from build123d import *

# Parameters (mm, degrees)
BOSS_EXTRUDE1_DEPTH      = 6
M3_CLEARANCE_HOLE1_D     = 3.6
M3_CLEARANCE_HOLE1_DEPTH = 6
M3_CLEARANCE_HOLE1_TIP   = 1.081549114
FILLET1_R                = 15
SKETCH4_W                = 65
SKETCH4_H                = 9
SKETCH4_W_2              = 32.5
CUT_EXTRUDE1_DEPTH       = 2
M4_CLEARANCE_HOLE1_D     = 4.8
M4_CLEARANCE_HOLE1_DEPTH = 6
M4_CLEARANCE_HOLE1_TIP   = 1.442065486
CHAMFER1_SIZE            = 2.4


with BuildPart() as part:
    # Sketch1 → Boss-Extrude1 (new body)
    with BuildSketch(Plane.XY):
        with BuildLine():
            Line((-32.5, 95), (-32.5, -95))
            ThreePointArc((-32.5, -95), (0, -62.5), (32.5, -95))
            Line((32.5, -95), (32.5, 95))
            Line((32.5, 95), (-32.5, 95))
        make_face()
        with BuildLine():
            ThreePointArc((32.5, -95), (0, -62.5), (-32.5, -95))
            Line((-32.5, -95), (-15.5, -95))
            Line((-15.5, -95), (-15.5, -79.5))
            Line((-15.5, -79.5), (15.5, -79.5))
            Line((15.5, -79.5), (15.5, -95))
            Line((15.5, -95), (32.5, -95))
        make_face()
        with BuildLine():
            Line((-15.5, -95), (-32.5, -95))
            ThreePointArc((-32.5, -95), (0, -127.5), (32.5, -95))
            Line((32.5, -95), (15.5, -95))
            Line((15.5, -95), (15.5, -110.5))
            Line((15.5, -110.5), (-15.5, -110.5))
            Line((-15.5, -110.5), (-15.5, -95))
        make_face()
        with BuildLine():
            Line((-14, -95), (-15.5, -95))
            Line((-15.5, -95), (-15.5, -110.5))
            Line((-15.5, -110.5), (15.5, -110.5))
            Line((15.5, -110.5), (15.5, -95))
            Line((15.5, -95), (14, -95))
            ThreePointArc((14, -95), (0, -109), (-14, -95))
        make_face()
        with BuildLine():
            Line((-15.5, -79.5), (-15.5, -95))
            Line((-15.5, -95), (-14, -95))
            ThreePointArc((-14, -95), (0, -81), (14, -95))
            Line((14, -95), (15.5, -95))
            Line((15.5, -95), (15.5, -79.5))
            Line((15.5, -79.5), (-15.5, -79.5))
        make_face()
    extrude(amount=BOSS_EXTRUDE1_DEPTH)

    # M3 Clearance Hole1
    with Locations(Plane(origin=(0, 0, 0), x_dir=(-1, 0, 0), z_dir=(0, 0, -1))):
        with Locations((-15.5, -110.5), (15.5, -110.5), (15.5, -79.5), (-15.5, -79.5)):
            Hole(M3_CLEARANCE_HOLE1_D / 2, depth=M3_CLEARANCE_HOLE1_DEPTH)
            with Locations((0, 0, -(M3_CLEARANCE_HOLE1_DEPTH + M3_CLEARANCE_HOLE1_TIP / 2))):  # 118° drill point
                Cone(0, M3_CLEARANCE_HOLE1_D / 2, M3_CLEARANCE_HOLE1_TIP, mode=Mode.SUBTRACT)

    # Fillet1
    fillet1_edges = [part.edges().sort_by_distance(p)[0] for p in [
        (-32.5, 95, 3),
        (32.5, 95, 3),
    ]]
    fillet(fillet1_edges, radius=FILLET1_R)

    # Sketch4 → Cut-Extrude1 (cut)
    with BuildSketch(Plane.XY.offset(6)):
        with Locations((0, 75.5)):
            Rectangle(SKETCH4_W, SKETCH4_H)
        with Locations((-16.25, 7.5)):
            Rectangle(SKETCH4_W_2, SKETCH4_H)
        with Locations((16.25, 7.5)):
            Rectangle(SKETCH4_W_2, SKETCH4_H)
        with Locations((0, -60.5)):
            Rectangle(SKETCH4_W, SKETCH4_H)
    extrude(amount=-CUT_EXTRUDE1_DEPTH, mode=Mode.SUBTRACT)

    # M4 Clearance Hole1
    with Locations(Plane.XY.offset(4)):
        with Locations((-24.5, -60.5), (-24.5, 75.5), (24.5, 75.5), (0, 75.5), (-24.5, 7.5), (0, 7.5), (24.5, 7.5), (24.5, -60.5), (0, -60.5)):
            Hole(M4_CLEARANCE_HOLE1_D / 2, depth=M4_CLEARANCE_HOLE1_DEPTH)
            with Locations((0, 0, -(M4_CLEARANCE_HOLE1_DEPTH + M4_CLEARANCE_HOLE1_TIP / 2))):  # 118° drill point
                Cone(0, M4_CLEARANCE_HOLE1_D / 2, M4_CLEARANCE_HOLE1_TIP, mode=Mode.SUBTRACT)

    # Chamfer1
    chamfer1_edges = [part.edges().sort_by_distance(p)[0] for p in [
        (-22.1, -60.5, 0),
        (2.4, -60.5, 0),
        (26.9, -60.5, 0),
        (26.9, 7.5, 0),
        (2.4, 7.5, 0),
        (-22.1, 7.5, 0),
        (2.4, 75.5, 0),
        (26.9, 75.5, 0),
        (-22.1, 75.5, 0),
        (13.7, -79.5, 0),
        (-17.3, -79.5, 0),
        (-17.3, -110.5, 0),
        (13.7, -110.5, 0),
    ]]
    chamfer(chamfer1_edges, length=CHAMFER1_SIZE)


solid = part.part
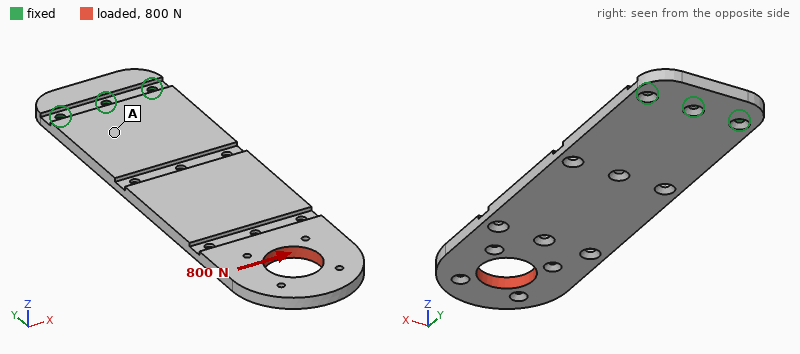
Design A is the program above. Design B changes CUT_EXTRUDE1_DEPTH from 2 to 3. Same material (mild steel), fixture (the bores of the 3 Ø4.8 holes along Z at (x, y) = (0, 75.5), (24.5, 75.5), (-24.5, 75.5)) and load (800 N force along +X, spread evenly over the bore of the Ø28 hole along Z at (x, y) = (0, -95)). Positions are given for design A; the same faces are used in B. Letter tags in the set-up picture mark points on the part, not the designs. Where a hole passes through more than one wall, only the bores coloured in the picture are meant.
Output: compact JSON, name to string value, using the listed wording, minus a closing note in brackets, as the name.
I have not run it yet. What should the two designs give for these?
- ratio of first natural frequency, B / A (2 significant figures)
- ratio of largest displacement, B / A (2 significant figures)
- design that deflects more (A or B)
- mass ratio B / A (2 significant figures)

{"ratio of first natural frequency, B / A": "0.72", "ratio of largest displacement, B / A": "1.3", "design that deflects more": "B", "mass ratio B / A": "0.98"}
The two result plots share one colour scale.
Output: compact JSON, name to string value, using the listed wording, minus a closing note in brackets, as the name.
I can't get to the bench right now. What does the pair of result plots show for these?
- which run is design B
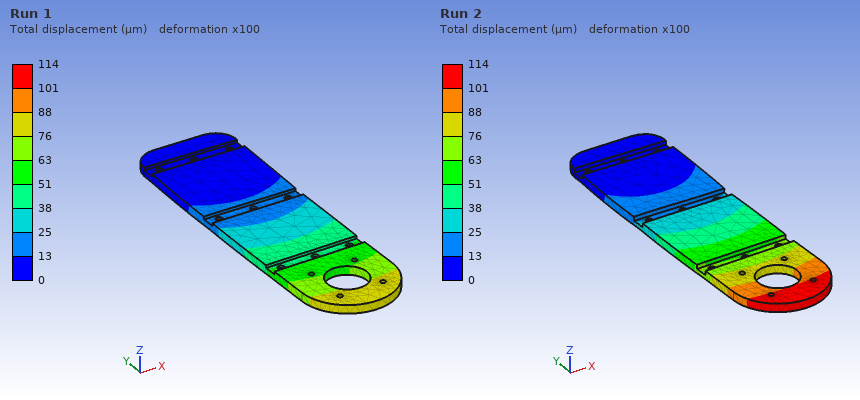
{"which run is design B": "Run 2"}
